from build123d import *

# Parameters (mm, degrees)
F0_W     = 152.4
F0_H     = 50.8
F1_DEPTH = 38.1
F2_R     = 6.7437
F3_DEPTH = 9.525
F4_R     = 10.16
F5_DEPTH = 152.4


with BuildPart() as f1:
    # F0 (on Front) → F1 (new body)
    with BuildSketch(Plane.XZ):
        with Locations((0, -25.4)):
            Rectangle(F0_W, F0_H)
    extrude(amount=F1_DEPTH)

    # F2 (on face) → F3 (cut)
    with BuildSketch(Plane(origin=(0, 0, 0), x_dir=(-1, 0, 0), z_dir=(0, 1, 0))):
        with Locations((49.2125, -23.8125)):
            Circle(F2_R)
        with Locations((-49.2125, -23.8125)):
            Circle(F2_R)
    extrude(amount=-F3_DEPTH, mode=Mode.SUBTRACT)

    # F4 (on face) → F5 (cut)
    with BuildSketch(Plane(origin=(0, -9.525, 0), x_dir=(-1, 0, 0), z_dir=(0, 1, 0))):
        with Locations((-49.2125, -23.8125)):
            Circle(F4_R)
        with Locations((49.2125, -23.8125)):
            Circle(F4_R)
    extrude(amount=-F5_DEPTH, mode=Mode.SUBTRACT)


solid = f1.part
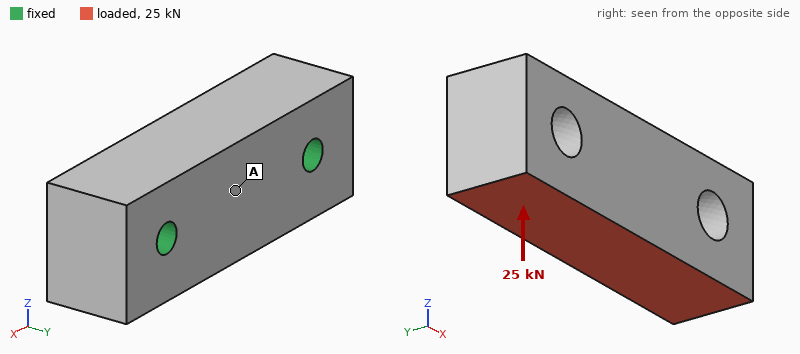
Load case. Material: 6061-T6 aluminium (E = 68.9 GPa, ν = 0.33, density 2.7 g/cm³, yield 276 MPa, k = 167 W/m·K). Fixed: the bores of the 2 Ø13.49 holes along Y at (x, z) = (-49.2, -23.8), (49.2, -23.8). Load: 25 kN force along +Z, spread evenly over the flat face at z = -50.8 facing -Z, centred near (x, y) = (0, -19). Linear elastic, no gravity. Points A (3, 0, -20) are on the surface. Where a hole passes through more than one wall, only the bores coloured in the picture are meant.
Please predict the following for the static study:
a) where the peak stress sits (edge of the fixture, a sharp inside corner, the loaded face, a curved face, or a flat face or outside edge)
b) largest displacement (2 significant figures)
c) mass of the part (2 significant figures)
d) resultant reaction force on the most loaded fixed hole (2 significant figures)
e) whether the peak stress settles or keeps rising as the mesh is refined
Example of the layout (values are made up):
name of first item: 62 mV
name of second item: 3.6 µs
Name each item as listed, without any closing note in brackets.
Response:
where the peak stress sits: edge of the fixture
largest displacement: 97 µm
mass of the part: 740 g
resultant reaction force on the most loaded fixed hole: 13 kN
whether the peak stress settles or keeps rising as the mesh is refined: keeps rising
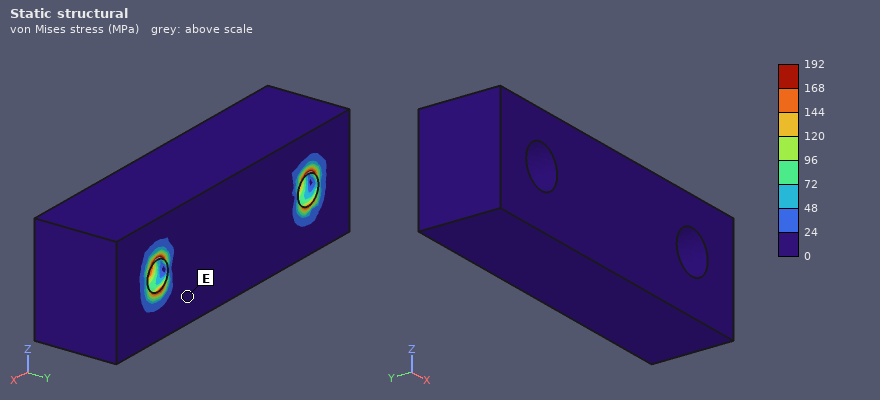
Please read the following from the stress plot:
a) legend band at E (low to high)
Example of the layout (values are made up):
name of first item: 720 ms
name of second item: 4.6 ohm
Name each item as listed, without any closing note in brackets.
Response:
legend band at E: 0 to 24 MPa
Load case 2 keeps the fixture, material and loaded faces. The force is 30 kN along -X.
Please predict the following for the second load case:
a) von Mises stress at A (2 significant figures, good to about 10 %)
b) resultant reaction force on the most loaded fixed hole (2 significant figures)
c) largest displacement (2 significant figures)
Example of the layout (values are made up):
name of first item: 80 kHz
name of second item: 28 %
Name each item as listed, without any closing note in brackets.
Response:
von Mises stress at A: 13 MPa
resultant reaction force on the most loaded fixed hole: 17 kN
largest displacement: 37 µm
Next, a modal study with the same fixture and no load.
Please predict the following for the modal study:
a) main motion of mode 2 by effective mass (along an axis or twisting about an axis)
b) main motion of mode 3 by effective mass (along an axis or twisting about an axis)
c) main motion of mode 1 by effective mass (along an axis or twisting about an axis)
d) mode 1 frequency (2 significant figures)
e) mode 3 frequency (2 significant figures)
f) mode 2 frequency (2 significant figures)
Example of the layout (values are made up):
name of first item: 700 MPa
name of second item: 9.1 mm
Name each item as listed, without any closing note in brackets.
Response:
main motion of mode 2 by effective mass: twisting about Y
main motion of mode 3 by effective mass: along Y
main motion of mode 1 by effective mass: along Z
mode 1 frequency: 3300 Hz
mode 3 frequency: 7700 Hz
mode 2 frequency: 7300 Hz
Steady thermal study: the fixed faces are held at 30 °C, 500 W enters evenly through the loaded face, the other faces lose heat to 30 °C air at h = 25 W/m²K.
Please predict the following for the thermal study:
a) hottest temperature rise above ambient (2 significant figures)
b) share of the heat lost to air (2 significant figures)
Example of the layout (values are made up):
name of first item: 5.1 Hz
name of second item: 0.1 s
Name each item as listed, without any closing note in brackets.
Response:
hottest temperature rise above ambient: 43 K
share of the heat lost to air: 3.5 %
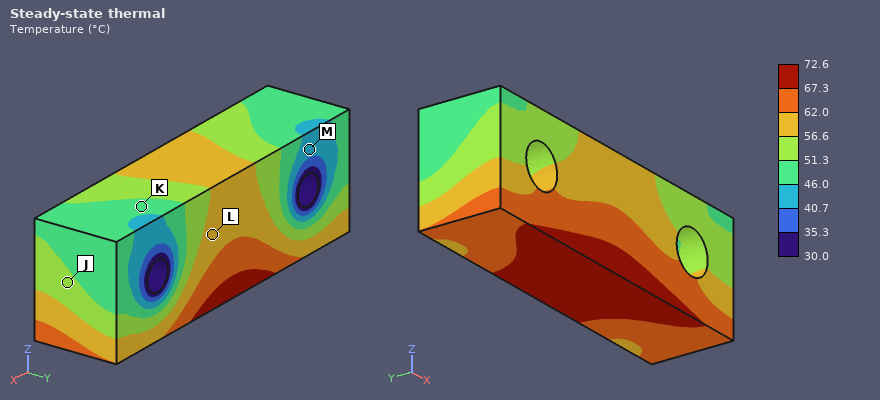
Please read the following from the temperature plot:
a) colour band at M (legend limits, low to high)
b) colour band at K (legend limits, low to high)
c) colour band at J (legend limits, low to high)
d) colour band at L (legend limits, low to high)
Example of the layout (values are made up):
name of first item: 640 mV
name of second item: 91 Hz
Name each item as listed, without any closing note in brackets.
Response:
colour band at M: 40.7 to 46.0 °C
colour band at K: 46.0 to 51.3 °C
colour band at J: 51.3 to 56.6 °C
colour band at L: 56.6 to 62.0 °C
